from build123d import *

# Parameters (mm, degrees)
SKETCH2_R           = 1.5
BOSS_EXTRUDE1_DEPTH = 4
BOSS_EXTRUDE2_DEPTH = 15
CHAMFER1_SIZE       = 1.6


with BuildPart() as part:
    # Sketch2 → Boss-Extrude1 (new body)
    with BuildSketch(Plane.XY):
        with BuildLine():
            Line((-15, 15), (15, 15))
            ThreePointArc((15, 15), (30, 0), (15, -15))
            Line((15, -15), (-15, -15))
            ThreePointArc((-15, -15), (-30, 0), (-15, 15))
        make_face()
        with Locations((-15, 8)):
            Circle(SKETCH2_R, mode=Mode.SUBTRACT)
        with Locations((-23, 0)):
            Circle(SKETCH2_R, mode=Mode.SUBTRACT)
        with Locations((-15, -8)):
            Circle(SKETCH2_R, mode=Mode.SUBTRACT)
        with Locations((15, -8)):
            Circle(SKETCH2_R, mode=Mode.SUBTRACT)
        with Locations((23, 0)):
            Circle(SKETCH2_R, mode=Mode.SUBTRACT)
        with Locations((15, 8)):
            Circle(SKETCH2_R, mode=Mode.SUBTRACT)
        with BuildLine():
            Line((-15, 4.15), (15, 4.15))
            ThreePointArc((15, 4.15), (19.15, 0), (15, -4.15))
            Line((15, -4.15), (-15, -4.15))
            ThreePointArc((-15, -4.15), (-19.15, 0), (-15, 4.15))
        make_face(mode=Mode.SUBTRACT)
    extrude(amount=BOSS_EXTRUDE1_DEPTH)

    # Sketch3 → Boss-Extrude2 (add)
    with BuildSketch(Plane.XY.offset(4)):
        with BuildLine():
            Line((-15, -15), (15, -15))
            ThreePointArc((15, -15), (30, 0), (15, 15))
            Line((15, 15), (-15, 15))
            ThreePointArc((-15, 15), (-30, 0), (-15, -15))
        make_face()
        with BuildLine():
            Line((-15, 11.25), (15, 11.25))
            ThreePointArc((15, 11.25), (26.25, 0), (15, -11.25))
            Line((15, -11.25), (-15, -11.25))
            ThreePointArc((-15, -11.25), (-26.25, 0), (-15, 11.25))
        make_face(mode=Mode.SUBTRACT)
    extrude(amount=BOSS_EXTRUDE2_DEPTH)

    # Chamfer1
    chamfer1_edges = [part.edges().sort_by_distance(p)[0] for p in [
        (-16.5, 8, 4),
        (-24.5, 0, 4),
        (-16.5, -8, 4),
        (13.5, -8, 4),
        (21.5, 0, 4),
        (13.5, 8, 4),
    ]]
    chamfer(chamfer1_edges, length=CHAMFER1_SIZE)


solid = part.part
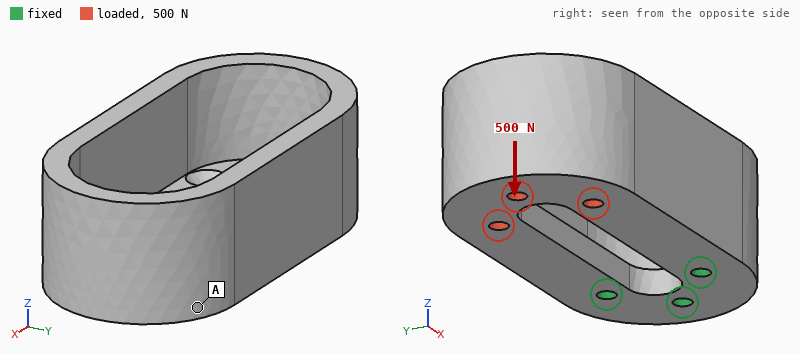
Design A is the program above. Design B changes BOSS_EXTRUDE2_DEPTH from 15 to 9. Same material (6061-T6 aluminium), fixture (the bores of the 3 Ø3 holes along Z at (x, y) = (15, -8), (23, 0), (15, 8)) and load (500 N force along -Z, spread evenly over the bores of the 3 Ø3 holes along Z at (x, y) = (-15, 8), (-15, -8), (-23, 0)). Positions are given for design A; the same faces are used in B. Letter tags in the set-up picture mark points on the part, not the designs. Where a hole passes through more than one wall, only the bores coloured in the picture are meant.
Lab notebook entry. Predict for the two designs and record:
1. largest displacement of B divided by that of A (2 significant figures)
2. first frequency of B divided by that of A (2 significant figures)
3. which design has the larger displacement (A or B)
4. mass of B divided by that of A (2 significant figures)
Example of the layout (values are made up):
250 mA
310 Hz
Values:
1.4
1.0
B
0.75
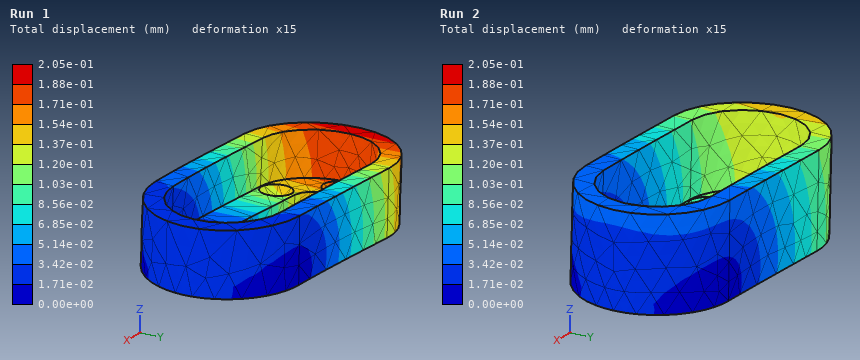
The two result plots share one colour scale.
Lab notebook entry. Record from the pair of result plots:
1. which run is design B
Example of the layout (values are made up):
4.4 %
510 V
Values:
Run 1
